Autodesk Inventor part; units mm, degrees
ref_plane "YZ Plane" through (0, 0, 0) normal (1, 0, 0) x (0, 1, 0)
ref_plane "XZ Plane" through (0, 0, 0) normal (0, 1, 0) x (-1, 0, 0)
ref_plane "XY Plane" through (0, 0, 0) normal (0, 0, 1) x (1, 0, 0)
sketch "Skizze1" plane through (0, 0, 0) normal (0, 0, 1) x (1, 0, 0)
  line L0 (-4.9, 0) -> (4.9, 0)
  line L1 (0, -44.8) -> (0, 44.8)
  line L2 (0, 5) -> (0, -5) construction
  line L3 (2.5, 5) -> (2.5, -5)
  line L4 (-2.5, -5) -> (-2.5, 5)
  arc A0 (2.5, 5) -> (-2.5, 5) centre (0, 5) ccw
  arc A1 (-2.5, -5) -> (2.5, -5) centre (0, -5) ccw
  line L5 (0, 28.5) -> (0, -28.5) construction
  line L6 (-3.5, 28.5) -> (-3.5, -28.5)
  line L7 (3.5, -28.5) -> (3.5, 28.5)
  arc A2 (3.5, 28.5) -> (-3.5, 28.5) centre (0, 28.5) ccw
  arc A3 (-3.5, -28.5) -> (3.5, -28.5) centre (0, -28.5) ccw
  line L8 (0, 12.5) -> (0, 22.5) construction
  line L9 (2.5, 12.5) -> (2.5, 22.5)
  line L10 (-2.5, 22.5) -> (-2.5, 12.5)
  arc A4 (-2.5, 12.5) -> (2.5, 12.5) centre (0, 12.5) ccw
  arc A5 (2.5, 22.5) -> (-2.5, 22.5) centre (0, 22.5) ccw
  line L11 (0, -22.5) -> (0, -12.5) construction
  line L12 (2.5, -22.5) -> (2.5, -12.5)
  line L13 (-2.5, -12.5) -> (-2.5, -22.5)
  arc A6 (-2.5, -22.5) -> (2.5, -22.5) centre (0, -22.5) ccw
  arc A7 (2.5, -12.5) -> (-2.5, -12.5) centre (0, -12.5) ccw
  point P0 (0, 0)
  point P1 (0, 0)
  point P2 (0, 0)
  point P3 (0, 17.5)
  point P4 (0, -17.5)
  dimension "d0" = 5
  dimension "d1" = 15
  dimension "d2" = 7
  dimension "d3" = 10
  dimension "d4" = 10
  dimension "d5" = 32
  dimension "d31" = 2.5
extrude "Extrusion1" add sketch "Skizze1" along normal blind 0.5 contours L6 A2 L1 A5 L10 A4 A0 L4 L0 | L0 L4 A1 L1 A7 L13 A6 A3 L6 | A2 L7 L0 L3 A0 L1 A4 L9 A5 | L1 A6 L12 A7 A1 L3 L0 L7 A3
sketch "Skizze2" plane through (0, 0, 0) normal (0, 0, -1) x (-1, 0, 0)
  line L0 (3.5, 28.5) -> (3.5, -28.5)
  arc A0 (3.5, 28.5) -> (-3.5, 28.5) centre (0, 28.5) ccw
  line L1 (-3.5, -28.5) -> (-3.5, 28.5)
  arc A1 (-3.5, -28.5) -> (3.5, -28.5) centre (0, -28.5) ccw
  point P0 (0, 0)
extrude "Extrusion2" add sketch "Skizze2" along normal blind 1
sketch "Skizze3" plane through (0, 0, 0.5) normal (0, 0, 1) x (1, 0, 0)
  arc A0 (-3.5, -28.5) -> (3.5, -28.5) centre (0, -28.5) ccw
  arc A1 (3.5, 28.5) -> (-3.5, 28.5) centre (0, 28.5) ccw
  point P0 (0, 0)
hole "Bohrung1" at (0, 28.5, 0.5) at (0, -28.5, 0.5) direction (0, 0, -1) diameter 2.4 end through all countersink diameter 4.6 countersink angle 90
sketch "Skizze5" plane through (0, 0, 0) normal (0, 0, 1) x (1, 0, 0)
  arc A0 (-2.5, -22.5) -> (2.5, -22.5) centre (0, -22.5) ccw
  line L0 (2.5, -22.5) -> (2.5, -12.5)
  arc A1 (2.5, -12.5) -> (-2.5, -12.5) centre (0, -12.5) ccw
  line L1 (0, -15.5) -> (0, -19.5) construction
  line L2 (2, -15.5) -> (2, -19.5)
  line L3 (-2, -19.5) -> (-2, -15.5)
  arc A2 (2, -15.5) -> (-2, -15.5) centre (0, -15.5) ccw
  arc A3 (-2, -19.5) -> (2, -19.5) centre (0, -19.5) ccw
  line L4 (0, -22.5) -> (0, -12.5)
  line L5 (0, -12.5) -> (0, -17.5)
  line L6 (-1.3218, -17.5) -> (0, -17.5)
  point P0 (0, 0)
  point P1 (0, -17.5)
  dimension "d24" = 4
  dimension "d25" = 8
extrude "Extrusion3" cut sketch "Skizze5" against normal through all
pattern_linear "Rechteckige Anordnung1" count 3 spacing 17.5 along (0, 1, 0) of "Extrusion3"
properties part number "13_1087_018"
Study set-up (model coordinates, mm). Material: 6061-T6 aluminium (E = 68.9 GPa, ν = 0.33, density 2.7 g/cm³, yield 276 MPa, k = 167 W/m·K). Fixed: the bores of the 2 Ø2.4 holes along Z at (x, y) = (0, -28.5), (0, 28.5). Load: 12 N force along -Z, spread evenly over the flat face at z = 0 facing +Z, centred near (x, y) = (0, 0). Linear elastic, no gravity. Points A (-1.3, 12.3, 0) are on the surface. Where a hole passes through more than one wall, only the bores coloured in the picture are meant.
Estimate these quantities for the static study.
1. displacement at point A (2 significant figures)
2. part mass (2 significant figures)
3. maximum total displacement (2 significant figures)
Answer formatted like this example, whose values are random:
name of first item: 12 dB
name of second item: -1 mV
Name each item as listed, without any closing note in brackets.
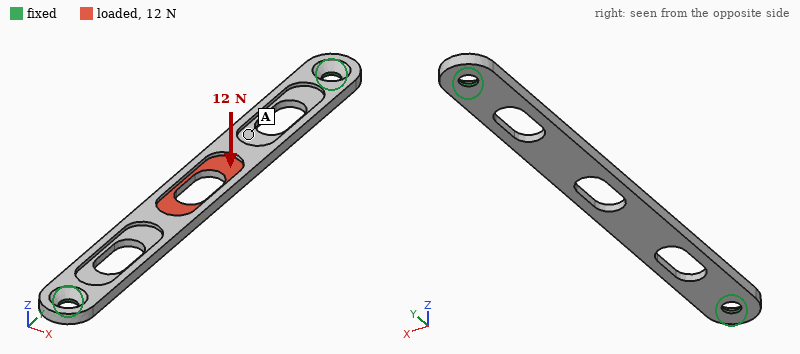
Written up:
displacement at point A: 0.094 mm
part mass: 1.2 g
maximum total displacement: 0.16 mm
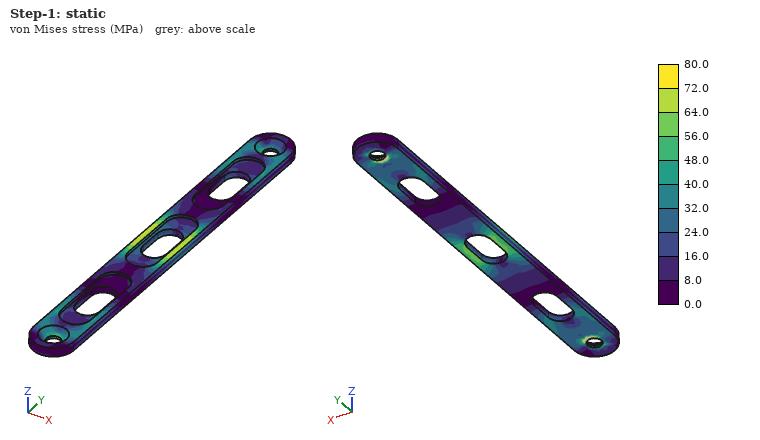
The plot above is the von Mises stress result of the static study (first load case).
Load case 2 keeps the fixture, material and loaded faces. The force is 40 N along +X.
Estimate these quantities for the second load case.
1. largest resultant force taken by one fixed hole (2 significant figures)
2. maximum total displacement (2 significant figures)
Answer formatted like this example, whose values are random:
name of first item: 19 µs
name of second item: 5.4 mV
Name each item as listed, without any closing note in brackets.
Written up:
largest resultant force taken by one fixed hole: 20 N
maximum total displacement: 49 µm
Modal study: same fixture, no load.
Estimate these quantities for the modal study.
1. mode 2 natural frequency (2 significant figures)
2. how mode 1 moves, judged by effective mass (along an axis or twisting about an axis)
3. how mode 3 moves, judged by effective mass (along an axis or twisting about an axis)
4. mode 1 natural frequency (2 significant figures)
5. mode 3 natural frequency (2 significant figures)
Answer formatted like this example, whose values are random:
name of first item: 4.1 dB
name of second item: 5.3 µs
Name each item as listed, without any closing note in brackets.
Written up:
mode 2 natural frequency: 5800 Hz
how mode 1 moves, judged by effective mass: along Z
how mode 3 moves, judged by effective mass: along X
mode 1 natural frequency: 2100 Hz
mode 3 natural frequency: 6300 Hz
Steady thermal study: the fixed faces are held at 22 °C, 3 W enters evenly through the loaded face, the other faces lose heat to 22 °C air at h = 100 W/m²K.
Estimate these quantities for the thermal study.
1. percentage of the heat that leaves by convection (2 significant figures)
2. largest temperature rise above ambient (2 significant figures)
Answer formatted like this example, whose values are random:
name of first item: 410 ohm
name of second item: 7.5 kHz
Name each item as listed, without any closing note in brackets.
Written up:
percentage of the heat that leaves by convection: 38 %
largest temperature rise above ambient: 24 K
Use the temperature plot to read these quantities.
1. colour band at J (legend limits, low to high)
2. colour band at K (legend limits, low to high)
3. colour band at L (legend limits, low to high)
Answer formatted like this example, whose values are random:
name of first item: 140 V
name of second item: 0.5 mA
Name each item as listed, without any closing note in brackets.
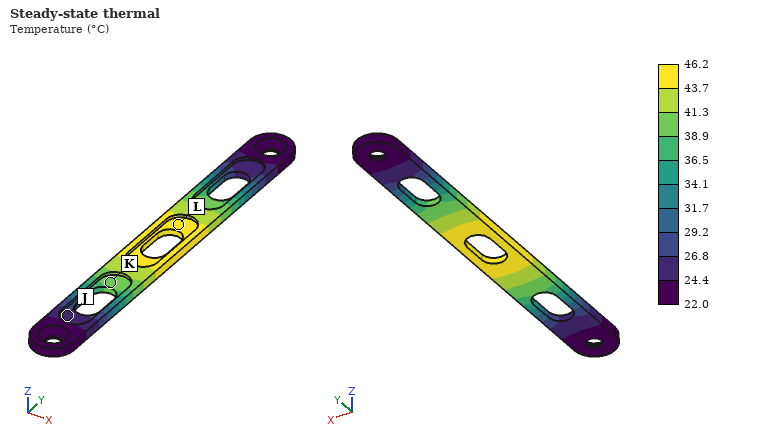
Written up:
colour band at J: 24.4 to 26.8 °C
colour band at K: 38.9 to 41.3 °C
colour band at L: 43.7 to 46.2 °C
